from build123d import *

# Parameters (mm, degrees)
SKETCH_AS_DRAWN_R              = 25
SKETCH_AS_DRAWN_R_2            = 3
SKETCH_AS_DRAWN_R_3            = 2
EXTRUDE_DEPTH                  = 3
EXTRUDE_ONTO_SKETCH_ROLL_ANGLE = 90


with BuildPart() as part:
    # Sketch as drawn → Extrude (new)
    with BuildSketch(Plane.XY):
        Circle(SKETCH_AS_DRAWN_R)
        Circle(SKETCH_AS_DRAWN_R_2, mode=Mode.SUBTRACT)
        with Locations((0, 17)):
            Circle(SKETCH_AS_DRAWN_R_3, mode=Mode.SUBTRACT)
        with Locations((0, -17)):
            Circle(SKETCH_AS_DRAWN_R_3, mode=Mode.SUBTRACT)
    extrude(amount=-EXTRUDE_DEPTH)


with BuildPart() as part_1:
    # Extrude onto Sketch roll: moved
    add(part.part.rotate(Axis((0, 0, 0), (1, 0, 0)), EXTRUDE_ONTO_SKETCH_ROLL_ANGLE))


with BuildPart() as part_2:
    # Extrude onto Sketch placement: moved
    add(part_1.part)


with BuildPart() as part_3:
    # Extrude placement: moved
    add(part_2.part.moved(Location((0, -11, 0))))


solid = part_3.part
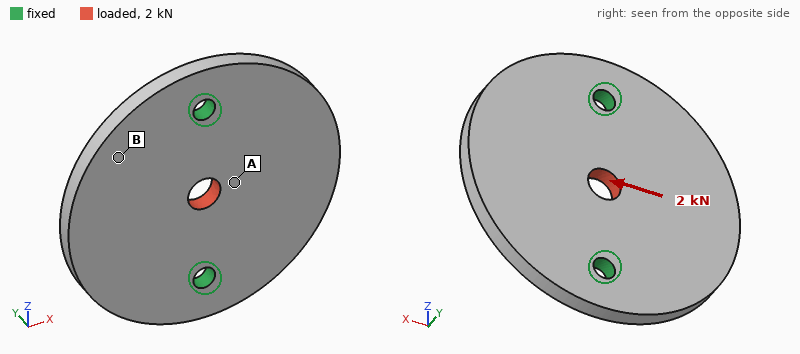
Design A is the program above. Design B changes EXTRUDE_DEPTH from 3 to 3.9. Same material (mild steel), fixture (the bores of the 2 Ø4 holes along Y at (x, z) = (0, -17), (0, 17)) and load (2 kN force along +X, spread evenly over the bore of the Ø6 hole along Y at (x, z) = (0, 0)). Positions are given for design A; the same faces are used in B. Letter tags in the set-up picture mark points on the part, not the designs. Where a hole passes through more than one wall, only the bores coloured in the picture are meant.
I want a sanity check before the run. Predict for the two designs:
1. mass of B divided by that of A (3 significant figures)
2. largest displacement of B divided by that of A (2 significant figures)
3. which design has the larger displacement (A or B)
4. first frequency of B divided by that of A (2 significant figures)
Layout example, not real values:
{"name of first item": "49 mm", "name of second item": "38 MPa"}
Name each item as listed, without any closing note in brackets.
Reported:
{"mass of B divided by that of A": "1.30", "largest displacement of B divided by that of A": "0.77", "which design has the larger displacement": "A", "first frequency of B divided by that of A": "1.3"}
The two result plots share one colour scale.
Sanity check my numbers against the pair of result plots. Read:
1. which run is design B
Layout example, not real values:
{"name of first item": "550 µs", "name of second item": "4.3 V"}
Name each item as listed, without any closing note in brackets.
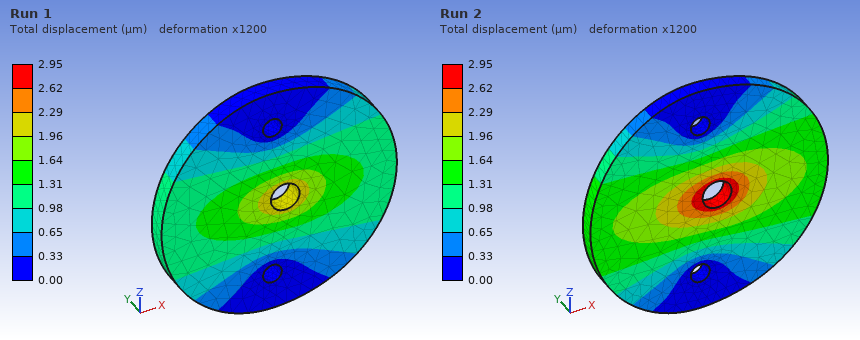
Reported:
{"which run is design B": "Run 1"}
